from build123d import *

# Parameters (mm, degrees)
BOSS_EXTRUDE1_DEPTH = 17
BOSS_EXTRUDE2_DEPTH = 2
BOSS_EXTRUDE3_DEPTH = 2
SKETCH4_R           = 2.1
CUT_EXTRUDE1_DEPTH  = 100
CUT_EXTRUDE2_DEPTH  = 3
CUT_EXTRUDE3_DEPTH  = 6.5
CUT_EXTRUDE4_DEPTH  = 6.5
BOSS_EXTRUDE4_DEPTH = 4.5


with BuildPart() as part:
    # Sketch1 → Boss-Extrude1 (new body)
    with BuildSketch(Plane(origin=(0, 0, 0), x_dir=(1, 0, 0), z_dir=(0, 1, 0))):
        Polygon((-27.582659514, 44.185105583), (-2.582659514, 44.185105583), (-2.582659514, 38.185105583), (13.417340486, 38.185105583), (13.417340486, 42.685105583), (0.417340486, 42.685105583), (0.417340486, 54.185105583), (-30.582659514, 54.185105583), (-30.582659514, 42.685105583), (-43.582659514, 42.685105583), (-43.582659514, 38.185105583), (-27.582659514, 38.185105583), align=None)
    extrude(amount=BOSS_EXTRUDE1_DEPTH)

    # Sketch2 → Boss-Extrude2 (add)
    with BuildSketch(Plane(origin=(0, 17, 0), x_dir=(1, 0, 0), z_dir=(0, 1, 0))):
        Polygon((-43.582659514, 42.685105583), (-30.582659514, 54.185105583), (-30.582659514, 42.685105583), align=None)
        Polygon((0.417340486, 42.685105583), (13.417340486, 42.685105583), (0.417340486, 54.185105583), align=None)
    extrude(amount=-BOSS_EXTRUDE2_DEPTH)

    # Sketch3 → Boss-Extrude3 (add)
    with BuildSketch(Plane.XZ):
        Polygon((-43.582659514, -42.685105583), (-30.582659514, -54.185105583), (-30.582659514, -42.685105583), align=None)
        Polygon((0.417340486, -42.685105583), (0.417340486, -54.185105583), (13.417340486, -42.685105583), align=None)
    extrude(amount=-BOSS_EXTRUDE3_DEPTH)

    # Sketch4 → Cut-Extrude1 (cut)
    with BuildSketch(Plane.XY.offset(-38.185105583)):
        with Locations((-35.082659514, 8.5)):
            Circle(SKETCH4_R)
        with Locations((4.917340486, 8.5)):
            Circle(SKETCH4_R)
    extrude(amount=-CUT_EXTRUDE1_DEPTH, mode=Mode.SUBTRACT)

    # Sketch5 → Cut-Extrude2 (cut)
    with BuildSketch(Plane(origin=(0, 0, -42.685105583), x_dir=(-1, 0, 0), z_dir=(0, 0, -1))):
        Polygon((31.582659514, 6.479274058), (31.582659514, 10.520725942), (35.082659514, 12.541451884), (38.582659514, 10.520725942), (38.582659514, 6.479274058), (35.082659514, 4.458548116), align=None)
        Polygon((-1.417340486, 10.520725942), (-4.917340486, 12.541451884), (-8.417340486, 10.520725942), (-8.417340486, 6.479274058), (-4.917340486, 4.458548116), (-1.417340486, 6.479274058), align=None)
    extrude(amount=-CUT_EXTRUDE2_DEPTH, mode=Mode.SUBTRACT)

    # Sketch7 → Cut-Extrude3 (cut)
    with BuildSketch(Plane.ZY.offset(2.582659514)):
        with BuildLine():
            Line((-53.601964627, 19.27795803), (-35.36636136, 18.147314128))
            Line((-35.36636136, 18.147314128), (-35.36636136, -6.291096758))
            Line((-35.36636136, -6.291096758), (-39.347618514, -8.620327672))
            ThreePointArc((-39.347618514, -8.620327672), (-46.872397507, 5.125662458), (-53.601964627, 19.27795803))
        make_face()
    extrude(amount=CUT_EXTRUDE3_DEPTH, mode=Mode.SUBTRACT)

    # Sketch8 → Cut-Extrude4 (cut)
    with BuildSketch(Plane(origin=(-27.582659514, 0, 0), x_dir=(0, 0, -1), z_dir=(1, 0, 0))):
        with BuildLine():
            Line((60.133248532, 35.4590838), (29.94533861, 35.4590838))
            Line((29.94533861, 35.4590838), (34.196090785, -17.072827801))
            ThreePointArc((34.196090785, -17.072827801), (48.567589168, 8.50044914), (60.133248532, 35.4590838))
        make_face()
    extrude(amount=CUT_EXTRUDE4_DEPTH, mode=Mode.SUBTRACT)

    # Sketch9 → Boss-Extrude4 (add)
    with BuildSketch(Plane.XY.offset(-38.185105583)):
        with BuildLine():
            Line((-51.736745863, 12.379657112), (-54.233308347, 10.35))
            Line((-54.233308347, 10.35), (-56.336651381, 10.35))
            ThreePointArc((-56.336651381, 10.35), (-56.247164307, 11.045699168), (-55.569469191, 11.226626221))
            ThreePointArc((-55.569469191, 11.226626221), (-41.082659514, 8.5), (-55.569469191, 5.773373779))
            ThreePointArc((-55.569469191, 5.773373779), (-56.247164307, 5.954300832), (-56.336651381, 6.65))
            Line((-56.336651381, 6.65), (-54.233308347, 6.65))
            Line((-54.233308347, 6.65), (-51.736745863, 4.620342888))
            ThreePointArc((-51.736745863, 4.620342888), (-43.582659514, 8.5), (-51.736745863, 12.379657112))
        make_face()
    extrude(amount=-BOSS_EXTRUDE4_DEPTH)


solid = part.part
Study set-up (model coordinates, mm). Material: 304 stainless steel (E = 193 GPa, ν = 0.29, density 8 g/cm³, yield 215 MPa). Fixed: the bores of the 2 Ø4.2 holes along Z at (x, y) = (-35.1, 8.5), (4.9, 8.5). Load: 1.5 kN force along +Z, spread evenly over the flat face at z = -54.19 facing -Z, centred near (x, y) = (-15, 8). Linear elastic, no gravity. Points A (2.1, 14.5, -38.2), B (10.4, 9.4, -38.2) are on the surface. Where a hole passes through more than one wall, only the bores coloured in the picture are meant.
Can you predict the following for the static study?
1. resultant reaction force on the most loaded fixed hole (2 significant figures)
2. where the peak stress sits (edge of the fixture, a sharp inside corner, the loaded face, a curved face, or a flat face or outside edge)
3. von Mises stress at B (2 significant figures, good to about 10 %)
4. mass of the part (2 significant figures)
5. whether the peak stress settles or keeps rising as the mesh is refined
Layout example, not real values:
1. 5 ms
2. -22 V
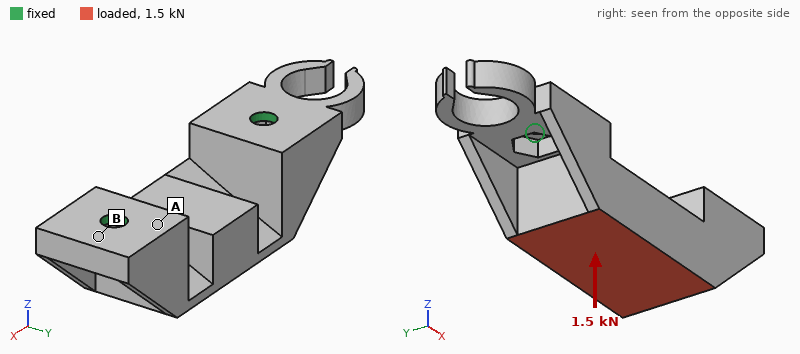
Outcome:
1. 880 N
2. edge of the fixture
3. 23 MPa
4. 60 g
5. keeps rising
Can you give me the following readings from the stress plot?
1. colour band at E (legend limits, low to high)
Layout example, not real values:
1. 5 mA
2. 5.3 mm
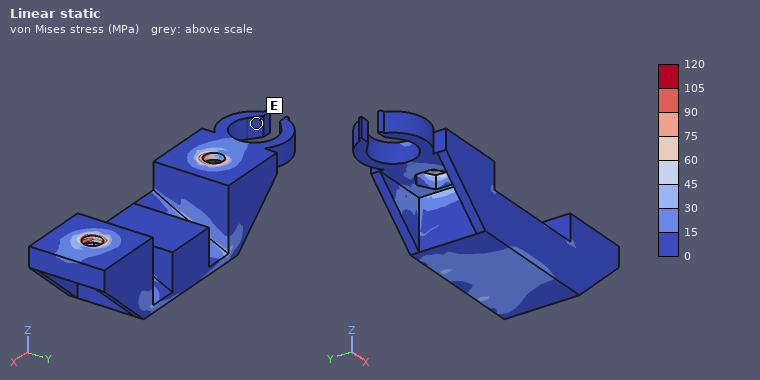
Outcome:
1. 0 to 15 MPa
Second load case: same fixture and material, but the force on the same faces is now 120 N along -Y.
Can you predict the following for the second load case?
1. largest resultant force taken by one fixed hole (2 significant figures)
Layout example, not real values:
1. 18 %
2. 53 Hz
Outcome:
1. 61 N
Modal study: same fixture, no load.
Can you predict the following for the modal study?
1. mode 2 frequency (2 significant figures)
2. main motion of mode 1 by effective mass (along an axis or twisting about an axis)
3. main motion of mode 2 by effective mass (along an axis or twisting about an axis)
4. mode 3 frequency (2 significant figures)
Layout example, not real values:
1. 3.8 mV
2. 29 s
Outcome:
1. 8300 Hz
2. along Y
3. along X
4. 9600 Hz
